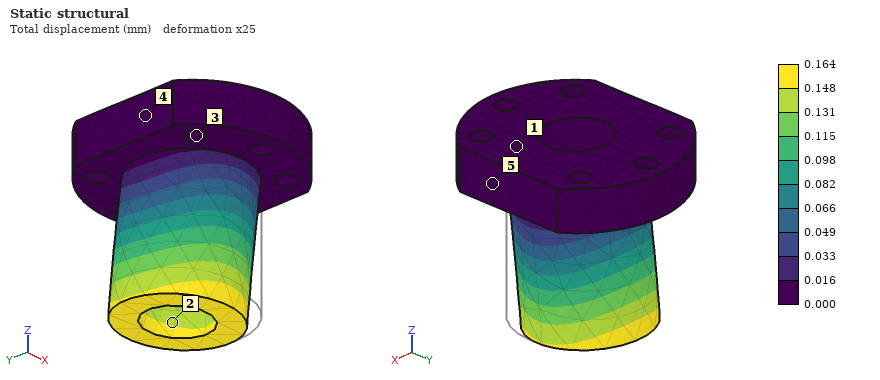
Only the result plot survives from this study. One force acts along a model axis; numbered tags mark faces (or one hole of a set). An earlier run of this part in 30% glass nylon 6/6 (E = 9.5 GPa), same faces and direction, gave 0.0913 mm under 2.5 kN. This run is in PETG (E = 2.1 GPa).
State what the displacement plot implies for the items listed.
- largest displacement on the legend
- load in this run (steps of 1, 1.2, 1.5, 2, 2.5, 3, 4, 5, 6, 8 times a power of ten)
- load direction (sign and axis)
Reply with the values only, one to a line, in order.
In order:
0.164 mm
1 kN
+Y
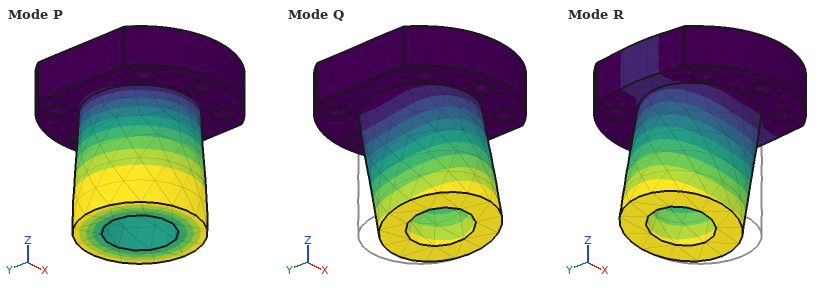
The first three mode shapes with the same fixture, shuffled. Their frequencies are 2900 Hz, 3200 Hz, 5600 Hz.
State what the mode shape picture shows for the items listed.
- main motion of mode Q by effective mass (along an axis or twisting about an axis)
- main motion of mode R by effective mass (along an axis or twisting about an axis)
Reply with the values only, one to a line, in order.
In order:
along Y
along X
